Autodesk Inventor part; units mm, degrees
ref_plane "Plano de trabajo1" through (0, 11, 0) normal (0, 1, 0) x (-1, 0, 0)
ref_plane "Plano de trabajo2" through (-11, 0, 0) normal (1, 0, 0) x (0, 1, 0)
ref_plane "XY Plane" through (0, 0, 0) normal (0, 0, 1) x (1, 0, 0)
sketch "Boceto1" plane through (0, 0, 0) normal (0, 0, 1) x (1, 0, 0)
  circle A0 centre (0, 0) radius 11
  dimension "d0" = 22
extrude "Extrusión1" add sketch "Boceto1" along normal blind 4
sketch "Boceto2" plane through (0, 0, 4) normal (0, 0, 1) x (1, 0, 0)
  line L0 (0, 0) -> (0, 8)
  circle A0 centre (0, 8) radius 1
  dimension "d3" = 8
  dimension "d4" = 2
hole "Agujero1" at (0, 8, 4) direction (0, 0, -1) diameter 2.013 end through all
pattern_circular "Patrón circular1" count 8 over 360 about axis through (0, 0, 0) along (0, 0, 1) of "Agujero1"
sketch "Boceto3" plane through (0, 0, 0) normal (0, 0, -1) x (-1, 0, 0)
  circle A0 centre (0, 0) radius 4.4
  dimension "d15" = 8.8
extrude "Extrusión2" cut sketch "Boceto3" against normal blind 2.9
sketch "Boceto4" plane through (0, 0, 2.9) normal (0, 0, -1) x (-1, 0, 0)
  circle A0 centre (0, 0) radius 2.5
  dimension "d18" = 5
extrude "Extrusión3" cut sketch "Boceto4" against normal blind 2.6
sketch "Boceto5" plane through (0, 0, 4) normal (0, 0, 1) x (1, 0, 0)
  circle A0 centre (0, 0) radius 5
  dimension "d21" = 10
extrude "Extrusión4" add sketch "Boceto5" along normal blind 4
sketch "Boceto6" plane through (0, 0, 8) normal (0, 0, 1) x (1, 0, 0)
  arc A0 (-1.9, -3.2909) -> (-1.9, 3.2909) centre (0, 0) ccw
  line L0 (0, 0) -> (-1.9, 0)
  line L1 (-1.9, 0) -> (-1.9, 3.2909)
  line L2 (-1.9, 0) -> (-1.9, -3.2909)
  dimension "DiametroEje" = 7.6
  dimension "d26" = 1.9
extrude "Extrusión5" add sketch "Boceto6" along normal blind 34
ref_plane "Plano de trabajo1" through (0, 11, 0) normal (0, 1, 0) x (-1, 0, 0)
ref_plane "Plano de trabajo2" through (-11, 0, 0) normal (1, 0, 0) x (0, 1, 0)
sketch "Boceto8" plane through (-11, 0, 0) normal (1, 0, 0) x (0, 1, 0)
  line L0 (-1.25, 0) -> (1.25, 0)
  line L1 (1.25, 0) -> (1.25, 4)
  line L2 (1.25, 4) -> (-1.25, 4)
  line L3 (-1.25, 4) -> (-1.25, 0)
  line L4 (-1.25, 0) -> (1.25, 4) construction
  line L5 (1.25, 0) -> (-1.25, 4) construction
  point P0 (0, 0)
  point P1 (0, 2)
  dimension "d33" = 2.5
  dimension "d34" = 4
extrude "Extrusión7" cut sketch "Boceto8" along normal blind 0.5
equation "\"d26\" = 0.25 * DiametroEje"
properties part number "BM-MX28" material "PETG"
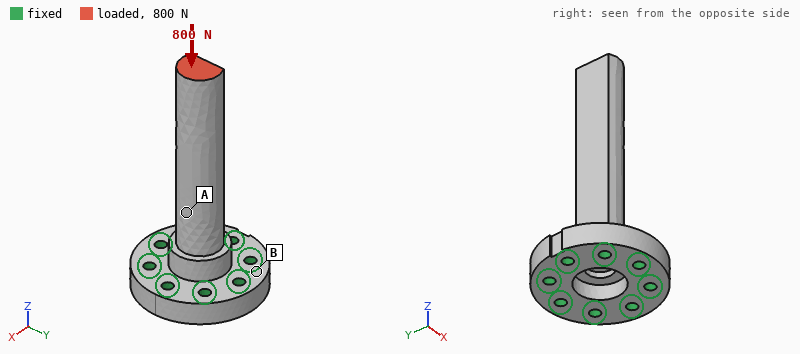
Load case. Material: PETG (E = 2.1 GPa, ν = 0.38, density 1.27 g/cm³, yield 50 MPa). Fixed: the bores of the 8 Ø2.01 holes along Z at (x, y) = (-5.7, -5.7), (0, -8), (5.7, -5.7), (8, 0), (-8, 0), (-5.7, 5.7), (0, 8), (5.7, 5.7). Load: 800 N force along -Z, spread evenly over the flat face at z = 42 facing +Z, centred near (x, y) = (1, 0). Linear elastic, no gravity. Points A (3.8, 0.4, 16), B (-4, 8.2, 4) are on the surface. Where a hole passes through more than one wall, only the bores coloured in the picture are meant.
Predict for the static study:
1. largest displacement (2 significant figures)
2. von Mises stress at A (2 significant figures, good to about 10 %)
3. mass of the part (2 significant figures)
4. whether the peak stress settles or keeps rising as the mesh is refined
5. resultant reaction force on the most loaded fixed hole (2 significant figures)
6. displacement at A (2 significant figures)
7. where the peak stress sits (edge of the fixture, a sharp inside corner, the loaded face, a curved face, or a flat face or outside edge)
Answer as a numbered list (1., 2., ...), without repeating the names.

1. 0.45 mm
2. 22 MPa
3. 3.5 g
4. keeps rising
5. 150 N
6. 0.17 mm
7. edge of the fixture
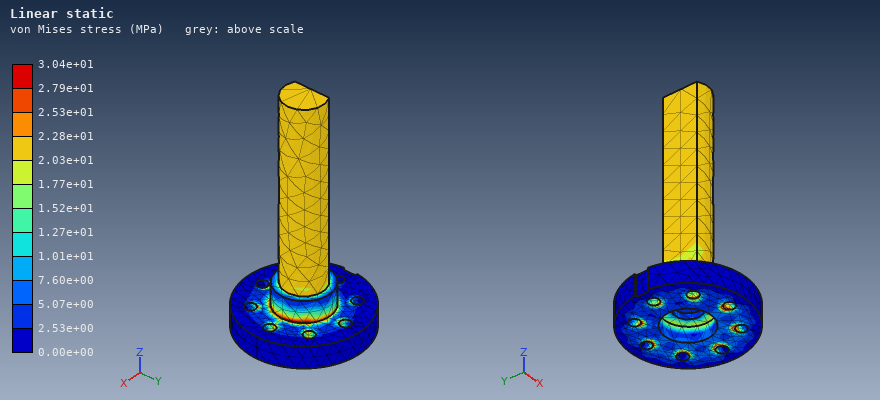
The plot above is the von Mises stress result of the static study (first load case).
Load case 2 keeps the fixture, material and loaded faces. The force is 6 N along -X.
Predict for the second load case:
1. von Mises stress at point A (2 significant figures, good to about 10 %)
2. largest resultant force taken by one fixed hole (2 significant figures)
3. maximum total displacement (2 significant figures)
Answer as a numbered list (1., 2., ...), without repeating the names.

1. 5.9 MPa
2. 11 N
3. 0.57 mm
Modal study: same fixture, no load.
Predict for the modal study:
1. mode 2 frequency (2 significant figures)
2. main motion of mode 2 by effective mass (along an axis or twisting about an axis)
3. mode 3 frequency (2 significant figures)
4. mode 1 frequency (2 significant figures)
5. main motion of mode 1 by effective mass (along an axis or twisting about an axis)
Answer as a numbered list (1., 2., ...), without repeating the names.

1. 1000 Hz
2. along Y
3. 4600 Hz
4. 810 Hz
5. along X
